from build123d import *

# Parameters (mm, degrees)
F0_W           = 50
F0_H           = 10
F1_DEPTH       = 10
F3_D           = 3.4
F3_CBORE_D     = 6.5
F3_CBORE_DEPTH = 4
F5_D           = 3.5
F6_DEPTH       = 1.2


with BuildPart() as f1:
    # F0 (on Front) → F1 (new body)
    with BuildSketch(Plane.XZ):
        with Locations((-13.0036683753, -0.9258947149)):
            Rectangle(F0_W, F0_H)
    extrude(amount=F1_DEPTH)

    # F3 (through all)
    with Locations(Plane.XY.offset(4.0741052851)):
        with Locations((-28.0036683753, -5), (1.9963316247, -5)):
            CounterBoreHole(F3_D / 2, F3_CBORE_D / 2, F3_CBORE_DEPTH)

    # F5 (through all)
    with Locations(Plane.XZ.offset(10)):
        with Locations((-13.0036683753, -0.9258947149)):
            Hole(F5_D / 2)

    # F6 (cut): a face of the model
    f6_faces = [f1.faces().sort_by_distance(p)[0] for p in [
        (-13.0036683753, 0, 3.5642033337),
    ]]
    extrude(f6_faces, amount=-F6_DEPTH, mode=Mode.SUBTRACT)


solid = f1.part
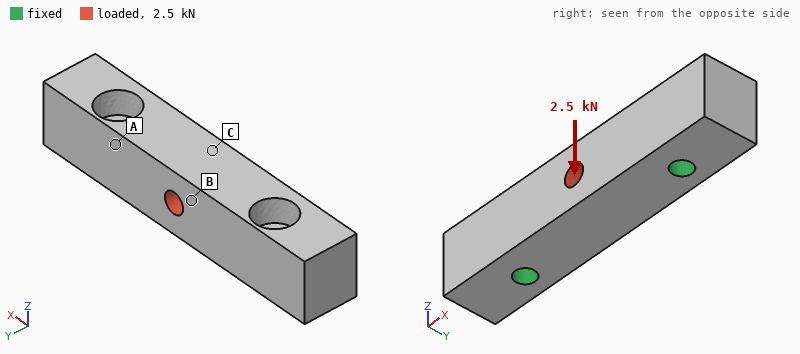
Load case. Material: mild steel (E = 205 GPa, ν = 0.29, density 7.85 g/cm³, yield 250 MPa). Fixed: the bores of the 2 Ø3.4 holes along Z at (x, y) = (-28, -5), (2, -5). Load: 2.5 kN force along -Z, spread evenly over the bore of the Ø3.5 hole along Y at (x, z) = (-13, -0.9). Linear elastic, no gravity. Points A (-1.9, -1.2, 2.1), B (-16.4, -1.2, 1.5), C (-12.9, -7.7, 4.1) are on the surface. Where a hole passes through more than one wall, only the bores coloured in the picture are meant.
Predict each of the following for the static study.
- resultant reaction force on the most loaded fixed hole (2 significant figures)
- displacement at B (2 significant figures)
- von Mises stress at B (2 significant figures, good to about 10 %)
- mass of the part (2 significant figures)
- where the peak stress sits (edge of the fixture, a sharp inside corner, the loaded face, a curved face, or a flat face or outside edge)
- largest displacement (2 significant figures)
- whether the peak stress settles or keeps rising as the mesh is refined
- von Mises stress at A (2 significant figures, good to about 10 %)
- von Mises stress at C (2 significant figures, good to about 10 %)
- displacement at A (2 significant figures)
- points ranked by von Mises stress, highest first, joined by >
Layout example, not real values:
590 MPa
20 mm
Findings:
1.4 kN
5.6 µm
45 MPa
31 g
edge of the fixture
7.0 µm
keeps rising
20 MPa
85 MPa
2.1 µm
C > B > A
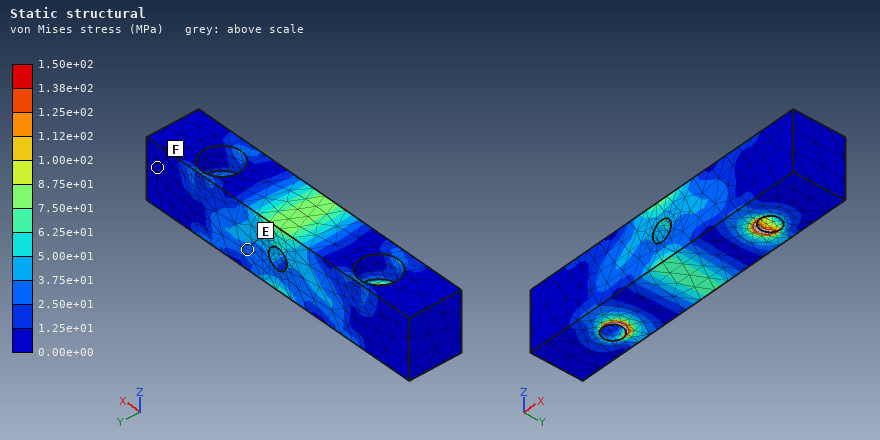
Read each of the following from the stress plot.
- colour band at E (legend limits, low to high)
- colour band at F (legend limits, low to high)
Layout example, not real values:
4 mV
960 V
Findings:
2.50e+01 to 3.75e+01 MPa
0.00e+00 to 1.25e+01 MPa
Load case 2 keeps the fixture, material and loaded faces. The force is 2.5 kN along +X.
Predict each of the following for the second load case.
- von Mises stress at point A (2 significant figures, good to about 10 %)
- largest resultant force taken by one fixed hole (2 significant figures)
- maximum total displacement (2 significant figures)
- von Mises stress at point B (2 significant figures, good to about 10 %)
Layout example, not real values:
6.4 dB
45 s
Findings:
13 MPa
1.3 kN
1.5 µm
17 MPa
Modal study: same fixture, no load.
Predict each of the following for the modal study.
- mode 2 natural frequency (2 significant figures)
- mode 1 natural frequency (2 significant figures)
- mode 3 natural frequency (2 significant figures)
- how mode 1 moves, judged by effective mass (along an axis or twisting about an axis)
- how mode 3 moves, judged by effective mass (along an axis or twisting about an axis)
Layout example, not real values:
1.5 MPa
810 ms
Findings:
32 kHz
26 kHz
35 kHz
along Y
along Y
